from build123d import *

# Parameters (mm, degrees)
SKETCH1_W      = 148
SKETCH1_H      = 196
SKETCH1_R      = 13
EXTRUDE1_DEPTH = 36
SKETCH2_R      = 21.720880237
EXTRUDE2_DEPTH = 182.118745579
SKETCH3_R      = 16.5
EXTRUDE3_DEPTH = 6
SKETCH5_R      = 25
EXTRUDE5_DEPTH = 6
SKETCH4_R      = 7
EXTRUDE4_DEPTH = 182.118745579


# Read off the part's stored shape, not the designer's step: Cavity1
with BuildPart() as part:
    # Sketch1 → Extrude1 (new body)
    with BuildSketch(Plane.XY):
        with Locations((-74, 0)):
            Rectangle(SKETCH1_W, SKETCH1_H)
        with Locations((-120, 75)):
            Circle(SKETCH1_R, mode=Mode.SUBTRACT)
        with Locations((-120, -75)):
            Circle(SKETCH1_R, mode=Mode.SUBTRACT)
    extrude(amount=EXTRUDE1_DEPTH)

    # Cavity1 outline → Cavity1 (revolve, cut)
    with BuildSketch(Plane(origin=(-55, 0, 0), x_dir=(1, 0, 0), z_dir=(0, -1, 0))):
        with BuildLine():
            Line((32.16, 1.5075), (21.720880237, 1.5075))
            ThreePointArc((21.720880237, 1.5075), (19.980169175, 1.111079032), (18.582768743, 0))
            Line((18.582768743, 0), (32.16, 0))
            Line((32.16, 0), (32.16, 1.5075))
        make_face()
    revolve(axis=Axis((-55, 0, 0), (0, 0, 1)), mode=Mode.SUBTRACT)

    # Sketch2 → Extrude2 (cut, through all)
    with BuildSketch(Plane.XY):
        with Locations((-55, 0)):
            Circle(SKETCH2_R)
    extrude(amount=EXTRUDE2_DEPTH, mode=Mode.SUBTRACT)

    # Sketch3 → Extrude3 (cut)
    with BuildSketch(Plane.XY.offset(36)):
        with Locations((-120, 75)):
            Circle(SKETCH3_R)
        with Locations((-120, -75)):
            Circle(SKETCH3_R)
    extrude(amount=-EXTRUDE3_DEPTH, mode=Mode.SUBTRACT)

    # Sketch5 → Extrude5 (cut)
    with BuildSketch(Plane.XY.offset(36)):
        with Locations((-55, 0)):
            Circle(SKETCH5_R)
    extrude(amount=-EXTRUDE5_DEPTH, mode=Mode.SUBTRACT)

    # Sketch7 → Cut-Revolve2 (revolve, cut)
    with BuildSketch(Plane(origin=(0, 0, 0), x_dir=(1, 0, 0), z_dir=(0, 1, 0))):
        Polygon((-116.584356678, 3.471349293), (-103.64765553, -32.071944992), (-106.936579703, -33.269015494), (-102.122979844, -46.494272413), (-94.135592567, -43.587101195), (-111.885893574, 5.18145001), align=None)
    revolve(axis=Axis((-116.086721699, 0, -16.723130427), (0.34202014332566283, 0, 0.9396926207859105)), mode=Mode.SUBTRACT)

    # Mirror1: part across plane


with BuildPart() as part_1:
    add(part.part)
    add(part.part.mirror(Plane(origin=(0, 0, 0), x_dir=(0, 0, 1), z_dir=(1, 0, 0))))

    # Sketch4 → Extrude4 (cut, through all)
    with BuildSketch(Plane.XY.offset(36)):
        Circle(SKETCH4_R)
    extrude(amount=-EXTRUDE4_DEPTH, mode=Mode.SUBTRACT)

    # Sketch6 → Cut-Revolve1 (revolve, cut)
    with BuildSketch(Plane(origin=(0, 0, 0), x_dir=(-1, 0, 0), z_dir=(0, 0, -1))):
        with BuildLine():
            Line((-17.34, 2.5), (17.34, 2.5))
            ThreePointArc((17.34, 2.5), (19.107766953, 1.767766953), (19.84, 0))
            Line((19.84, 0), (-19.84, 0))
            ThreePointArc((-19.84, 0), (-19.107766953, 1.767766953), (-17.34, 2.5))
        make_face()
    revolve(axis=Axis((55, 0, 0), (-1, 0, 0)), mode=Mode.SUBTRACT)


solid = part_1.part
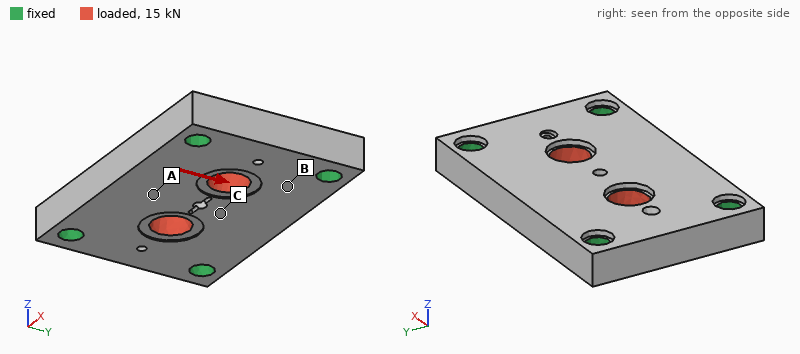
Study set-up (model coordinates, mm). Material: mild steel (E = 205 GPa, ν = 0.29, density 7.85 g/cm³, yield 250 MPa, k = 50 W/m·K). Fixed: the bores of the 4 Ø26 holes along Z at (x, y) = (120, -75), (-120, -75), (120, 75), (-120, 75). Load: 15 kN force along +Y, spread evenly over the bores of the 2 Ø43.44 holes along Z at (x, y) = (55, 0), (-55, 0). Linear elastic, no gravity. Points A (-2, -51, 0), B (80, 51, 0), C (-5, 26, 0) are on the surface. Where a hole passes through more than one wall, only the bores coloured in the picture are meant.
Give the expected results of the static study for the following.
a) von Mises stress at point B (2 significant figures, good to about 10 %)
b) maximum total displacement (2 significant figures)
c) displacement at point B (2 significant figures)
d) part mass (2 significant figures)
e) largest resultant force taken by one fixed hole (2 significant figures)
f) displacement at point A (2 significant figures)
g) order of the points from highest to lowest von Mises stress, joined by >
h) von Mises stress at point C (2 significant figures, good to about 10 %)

2.5 MPa
1.8 µm
0.72 µm
15 kg
4.3 kN
1.6 µm
B > C > A
0.98 MPa
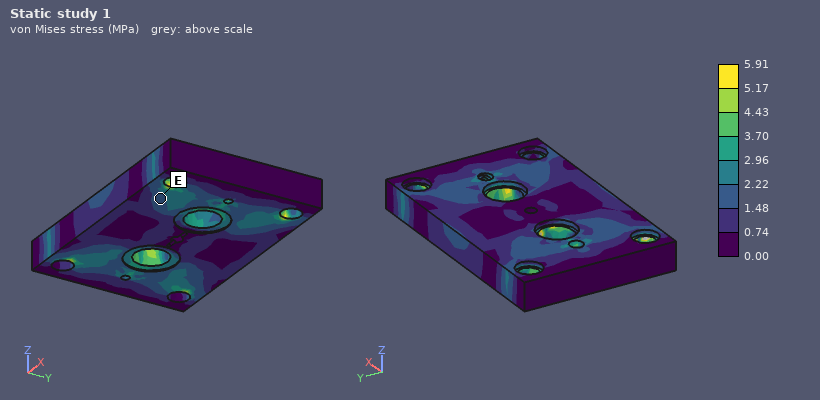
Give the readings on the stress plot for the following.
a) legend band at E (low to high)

1.48 to 2.22 MPa
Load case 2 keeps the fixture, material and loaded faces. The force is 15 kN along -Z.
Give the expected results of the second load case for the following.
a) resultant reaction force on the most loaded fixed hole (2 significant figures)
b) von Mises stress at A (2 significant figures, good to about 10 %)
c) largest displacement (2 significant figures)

3.8 kN
3.8 MPa
10 µm
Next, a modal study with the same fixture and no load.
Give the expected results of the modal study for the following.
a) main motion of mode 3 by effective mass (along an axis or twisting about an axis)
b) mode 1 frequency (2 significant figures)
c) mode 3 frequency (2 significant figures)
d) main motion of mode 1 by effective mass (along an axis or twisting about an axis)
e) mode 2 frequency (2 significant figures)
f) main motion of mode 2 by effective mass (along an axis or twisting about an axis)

along Y
2600 Hz
5300 Hz
along Z
3600 Hz
twisting about X
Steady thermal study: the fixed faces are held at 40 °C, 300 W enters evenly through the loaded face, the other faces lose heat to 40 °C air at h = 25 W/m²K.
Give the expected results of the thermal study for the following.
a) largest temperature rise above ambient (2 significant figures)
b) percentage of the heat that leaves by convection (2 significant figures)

44 K
21 %
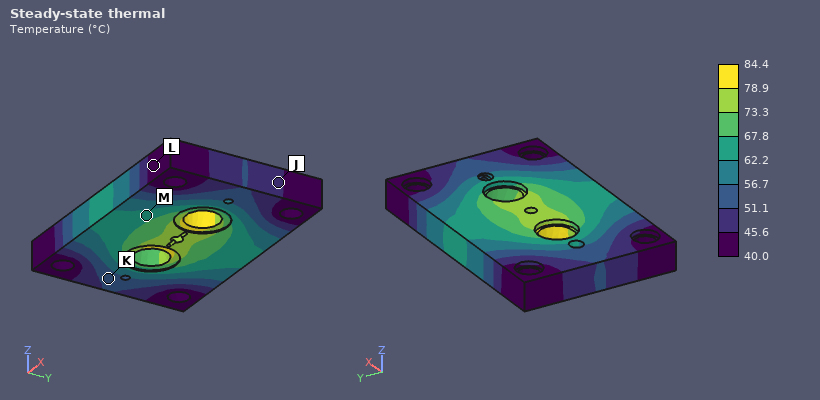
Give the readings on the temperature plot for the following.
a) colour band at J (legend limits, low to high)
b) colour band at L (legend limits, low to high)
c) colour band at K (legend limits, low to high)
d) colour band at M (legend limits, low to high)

45.6 to 51.1 °C
40.0 to 45.6 °C
51.1 to 56.7 °C
62.2 to 67.8 °C
